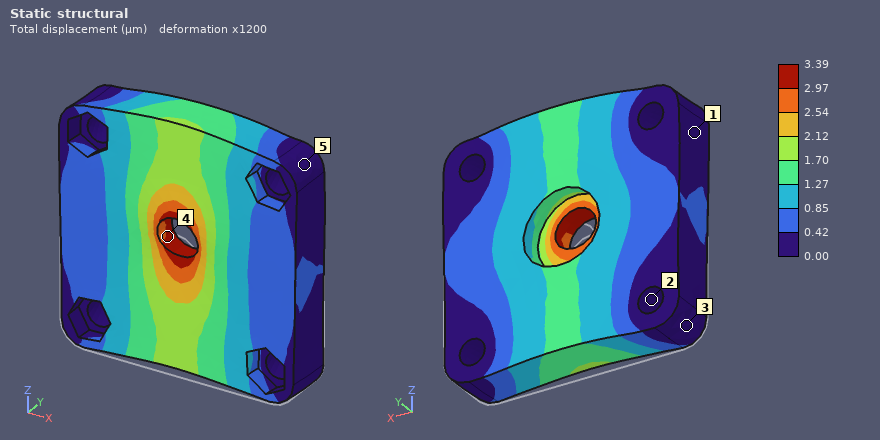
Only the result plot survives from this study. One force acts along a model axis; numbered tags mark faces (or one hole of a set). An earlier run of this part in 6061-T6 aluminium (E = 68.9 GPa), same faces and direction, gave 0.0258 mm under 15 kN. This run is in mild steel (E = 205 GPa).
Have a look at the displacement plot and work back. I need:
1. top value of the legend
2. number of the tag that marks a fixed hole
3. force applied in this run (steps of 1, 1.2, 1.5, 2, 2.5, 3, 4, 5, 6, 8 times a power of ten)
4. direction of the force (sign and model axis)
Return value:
3.39 µm
2
6 kN
+Z
